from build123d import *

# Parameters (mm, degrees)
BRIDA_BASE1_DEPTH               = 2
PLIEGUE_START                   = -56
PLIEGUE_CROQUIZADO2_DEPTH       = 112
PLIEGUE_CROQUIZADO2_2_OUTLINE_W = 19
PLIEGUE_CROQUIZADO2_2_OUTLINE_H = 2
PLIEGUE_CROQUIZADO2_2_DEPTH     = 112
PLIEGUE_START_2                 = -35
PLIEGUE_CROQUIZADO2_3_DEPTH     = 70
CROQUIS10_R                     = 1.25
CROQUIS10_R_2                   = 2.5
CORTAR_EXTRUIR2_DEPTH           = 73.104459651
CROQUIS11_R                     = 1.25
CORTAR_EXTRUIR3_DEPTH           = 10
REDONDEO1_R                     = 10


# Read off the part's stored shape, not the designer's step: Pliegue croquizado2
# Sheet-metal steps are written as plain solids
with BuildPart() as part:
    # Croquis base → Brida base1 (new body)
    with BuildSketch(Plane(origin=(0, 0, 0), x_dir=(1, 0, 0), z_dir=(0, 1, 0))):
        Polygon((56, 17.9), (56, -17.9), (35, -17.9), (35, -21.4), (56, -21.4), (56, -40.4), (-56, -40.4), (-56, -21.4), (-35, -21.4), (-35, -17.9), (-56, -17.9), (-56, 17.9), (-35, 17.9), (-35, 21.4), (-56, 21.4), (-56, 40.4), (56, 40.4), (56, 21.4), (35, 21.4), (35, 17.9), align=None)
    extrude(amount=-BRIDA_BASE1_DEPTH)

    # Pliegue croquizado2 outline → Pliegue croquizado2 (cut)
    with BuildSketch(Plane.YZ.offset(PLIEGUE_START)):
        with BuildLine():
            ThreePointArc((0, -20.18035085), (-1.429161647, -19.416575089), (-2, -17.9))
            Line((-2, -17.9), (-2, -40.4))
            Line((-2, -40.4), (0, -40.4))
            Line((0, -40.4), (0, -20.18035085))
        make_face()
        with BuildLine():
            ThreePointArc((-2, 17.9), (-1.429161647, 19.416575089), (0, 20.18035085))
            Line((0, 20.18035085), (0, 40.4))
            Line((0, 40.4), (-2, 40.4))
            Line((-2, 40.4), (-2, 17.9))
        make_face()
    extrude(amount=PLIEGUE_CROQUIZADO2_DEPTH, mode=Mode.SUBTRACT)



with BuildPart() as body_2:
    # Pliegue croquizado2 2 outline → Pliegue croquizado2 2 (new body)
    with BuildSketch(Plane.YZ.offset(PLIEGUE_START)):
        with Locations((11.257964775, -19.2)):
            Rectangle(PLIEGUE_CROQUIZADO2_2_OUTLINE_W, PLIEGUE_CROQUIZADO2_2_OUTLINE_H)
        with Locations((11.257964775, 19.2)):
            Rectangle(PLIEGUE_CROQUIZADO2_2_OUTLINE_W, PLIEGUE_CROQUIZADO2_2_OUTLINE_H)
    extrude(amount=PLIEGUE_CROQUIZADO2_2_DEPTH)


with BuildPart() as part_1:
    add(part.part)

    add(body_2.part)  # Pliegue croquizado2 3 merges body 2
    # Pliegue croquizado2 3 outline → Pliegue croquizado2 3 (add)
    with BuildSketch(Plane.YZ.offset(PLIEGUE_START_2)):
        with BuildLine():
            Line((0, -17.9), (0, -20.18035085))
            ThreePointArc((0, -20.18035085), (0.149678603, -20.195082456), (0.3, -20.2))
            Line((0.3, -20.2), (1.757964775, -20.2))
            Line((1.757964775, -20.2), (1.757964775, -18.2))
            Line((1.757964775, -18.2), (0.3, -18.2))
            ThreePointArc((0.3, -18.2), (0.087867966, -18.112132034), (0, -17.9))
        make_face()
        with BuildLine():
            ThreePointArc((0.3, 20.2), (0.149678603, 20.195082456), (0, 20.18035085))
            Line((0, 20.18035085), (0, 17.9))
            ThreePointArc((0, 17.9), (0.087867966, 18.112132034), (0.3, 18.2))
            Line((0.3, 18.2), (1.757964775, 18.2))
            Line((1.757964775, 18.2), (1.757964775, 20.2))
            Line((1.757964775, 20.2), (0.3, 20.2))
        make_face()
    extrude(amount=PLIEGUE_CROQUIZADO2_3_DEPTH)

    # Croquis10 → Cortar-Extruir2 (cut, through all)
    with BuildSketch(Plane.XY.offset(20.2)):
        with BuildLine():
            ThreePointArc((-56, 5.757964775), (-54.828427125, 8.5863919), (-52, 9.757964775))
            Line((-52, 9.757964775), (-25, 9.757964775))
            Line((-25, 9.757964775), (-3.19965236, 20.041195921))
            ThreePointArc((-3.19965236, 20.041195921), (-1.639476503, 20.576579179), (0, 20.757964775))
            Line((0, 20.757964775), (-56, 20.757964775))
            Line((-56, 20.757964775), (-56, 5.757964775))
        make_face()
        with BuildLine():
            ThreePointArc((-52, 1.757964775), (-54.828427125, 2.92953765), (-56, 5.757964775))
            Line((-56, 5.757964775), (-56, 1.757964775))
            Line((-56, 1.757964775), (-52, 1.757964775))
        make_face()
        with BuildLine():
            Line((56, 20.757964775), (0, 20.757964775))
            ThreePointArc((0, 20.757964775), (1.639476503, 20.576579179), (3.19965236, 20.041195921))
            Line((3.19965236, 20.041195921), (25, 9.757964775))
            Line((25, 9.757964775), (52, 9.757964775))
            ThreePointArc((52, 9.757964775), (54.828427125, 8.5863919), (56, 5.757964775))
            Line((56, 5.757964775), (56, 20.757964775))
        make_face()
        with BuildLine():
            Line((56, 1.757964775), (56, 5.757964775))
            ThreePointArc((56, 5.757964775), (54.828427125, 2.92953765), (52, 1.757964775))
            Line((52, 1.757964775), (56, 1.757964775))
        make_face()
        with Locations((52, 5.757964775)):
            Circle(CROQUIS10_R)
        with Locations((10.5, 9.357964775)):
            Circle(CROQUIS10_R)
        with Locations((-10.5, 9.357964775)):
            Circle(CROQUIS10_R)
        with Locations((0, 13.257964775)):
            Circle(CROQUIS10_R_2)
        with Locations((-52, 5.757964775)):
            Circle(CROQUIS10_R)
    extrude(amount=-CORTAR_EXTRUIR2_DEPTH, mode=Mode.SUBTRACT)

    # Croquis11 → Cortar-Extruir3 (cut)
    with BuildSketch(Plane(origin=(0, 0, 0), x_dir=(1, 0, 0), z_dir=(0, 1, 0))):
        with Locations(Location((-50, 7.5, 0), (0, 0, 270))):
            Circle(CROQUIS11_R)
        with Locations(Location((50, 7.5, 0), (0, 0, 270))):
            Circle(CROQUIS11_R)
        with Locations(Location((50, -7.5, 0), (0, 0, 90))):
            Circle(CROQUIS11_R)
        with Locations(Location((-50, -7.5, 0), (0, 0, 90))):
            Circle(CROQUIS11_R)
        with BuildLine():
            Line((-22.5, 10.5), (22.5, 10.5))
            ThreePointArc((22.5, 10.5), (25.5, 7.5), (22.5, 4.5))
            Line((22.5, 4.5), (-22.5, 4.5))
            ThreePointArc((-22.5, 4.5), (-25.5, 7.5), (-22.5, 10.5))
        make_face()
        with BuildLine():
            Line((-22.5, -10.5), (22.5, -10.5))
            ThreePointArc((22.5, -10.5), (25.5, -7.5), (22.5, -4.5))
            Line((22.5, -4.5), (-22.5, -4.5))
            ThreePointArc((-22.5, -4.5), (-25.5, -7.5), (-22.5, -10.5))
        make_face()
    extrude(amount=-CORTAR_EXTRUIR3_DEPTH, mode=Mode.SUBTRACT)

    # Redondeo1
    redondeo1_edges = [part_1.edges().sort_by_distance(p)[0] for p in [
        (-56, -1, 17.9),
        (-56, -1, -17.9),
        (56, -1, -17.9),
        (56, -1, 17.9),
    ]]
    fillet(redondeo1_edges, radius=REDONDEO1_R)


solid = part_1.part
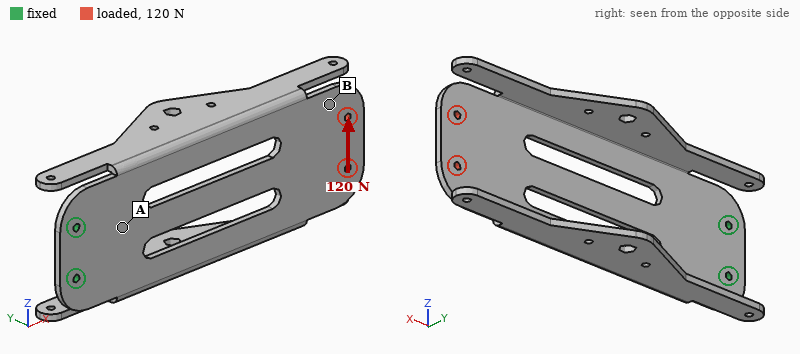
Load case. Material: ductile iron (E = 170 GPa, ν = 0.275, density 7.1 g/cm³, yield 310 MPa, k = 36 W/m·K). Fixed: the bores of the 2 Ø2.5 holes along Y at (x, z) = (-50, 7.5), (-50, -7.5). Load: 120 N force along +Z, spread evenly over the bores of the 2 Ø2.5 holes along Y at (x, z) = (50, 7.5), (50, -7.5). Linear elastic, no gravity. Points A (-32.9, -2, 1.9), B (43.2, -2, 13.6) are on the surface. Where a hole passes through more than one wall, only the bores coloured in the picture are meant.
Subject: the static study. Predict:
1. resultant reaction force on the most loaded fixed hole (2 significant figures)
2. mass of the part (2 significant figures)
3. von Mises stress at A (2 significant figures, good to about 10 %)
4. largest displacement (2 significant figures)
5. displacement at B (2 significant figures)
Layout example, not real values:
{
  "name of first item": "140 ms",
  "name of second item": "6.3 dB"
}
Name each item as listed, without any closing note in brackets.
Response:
{
  "resultant reaction force on the most loaded fixed hole": "720 N",
  "mass of the part": "86 g",
  "von Mises stress at A": "16 MPa",
  "largest displacement": "71 µm",
  "displacement at B": "63 µm"
}
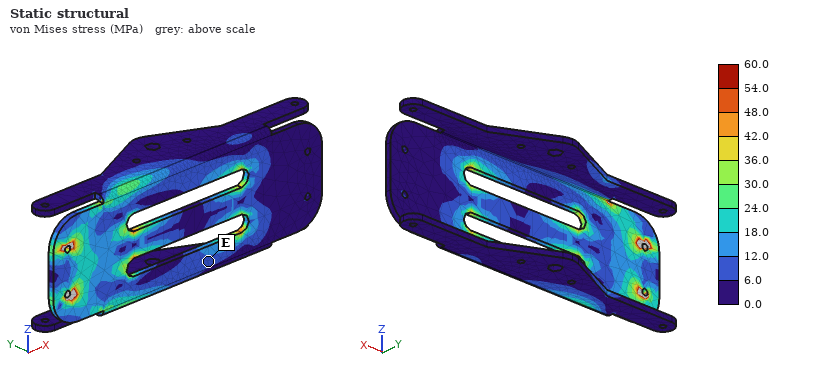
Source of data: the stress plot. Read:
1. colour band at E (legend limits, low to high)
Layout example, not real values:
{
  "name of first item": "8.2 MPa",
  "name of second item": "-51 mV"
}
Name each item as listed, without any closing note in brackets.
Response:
{
  "colour band at E": "6.0 to 12.0 MPa"
}
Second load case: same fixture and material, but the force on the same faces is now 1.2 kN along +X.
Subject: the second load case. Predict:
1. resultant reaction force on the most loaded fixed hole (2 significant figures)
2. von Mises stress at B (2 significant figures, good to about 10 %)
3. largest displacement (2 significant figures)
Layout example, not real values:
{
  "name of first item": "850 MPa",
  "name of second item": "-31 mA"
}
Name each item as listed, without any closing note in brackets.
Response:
{
  "resultant reaction force on the most loaded fixed hole": "600 N",
  "von Mises stress at B": "18 MPa",
  "largest displacement": "35 µm"
}
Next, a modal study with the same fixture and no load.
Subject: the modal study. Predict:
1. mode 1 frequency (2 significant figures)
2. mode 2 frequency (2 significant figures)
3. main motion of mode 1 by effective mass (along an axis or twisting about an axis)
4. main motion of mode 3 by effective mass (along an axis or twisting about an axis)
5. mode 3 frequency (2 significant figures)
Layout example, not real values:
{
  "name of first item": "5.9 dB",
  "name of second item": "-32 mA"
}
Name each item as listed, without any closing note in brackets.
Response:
{
  "mode 1 frequency": "140 Hz",
  "mode 2 frequency": "490 Hz",
  "main motion of mode 1 by effective mass": "along Y",
  "main motion of mode 3 by effective mass": "along Z",
  "mode 3 frequency": "1200 Hz"
}
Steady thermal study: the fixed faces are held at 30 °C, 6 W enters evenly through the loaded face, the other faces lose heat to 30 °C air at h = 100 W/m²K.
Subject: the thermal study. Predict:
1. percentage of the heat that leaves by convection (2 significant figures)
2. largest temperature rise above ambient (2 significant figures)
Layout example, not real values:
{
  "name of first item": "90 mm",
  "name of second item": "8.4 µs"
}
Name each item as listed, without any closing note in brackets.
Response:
{
  "percentage of the heat that leaves by convection": "100 %",
  "largest temperature rise above ambient": "40 K"
}
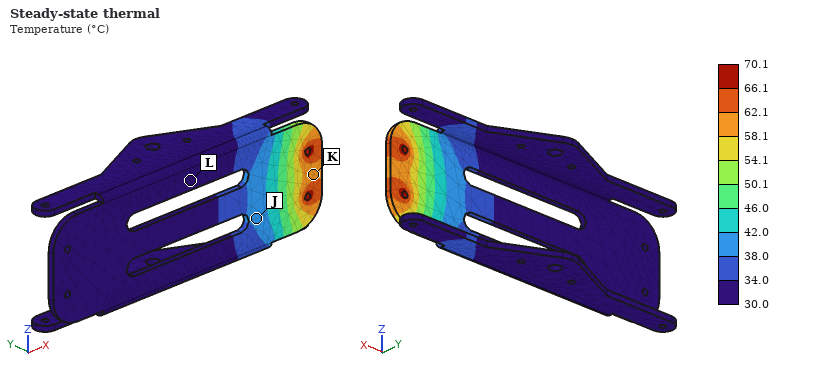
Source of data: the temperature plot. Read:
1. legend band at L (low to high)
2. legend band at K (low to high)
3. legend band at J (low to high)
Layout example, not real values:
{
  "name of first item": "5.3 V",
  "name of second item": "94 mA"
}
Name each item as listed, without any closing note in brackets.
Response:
{
  "legend band at L": "30.0 to 34.0 °C",
  "legend band at K": "58.1 to 62.1 °C",
  "legend band at J": "38.0 to 42.0 °C"
}
